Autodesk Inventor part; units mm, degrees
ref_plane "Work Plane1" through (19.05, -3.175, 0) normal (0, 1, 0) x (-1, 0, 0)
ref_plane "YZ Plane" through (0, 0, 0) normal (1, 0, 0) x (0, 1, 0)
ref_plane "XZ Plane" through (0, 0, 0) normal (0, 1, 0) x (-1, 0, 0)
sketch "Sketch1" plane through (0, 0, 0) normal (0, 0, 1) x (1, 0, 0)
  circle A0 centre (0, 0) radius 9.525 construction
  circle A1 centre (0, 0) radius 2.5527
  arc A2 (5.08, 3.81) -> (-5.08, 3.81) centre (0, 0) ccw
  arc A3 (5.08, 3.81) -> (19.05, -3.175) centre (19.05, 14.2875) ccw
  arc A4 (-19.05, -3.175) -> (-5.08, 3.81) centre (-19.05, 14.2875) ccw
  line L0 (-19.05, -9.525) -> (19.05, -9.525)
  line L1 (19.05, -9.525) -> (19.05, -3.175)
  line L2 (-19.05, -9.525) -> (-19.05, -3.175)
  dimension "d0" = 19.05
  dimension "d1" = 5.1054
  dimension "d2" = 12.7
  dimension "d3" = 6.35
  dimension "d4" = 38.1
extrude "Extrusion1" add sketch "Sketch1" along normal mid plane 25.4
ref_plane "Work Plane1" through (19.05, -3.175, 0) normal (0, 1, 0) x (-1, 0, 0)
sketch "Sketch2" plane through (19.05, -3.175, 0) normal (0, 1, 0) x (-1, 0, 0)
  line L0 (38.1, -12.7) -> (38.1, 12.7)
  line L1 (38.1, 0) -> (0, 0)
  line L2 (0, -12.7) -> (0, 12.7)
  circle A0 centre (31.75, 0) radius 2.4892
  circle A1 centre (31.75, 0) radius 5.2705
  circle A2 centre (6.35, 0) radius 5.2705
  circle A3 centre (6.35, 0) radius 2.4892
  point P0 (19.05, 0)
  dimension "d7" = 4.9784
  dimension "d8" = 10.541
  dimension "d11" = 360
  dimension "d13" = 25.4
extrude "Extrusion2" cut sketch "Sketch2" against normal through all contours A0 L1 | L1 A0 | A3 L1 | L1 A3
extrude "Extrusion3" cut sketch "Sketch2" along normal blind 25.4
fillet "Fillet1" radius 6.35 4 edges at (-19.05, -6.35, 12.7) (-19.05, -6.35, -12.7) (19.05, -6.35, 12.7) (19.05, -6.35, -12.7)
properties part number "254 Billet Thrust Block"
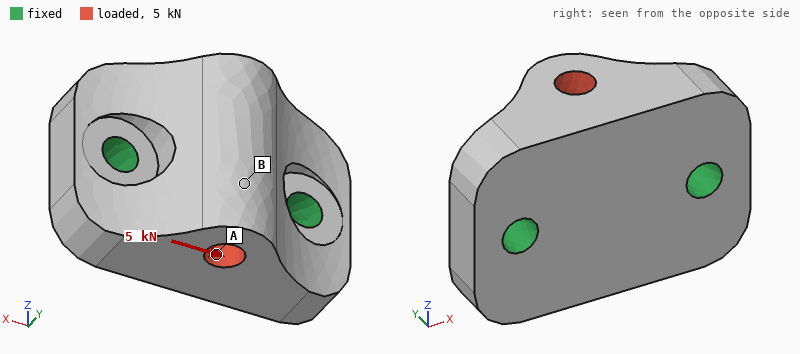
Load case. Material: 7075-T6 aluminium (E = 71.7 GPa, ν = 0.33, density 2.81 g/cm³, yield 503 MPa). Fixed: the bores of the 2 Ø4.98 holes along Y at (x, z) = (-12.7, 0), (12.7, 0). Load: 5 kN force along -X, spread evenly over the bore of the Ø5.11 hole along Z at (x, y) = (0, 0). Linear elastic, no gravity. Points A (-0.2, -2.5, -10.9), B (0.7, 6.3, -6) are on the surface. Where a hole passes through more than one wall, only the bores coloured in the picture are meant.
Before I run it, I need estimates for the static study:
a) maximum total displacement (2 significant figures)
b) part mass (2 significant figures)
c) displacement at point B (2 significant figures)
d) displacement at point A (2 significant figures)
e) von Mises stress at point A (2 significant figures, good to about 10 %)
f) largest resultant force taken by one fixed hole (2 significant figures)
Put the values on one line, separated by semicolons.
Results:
8.2 µm; 24 g; 7.8 µm; 4.6 µm; 23 MPa; 2.8 kN
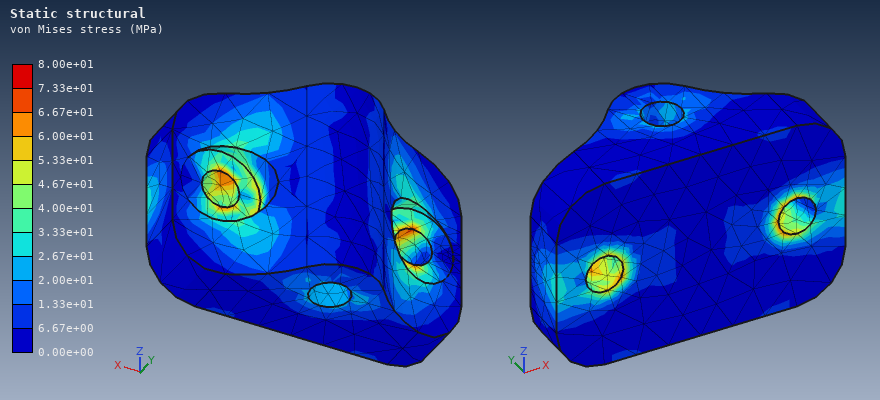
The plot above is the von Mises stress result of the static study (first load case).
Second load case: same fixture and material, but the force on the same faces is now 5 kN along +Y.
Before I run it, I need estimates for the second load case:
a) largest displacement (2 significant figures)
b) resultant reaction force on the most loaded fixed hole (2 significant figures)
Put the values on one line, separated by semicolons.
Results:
13 µm; 2.7 kN
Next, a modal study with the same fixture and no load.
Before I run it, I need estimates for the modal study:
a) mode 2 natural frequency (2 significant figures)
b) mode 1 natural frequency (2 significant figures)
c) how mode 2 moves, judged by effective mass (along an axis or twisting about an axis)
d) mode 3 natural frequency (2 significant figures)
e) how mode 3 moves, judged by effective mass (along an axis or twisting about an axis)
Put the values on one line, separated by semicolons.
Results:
28 kHz; 17 kHz; along Y; 38 kHz; along X
